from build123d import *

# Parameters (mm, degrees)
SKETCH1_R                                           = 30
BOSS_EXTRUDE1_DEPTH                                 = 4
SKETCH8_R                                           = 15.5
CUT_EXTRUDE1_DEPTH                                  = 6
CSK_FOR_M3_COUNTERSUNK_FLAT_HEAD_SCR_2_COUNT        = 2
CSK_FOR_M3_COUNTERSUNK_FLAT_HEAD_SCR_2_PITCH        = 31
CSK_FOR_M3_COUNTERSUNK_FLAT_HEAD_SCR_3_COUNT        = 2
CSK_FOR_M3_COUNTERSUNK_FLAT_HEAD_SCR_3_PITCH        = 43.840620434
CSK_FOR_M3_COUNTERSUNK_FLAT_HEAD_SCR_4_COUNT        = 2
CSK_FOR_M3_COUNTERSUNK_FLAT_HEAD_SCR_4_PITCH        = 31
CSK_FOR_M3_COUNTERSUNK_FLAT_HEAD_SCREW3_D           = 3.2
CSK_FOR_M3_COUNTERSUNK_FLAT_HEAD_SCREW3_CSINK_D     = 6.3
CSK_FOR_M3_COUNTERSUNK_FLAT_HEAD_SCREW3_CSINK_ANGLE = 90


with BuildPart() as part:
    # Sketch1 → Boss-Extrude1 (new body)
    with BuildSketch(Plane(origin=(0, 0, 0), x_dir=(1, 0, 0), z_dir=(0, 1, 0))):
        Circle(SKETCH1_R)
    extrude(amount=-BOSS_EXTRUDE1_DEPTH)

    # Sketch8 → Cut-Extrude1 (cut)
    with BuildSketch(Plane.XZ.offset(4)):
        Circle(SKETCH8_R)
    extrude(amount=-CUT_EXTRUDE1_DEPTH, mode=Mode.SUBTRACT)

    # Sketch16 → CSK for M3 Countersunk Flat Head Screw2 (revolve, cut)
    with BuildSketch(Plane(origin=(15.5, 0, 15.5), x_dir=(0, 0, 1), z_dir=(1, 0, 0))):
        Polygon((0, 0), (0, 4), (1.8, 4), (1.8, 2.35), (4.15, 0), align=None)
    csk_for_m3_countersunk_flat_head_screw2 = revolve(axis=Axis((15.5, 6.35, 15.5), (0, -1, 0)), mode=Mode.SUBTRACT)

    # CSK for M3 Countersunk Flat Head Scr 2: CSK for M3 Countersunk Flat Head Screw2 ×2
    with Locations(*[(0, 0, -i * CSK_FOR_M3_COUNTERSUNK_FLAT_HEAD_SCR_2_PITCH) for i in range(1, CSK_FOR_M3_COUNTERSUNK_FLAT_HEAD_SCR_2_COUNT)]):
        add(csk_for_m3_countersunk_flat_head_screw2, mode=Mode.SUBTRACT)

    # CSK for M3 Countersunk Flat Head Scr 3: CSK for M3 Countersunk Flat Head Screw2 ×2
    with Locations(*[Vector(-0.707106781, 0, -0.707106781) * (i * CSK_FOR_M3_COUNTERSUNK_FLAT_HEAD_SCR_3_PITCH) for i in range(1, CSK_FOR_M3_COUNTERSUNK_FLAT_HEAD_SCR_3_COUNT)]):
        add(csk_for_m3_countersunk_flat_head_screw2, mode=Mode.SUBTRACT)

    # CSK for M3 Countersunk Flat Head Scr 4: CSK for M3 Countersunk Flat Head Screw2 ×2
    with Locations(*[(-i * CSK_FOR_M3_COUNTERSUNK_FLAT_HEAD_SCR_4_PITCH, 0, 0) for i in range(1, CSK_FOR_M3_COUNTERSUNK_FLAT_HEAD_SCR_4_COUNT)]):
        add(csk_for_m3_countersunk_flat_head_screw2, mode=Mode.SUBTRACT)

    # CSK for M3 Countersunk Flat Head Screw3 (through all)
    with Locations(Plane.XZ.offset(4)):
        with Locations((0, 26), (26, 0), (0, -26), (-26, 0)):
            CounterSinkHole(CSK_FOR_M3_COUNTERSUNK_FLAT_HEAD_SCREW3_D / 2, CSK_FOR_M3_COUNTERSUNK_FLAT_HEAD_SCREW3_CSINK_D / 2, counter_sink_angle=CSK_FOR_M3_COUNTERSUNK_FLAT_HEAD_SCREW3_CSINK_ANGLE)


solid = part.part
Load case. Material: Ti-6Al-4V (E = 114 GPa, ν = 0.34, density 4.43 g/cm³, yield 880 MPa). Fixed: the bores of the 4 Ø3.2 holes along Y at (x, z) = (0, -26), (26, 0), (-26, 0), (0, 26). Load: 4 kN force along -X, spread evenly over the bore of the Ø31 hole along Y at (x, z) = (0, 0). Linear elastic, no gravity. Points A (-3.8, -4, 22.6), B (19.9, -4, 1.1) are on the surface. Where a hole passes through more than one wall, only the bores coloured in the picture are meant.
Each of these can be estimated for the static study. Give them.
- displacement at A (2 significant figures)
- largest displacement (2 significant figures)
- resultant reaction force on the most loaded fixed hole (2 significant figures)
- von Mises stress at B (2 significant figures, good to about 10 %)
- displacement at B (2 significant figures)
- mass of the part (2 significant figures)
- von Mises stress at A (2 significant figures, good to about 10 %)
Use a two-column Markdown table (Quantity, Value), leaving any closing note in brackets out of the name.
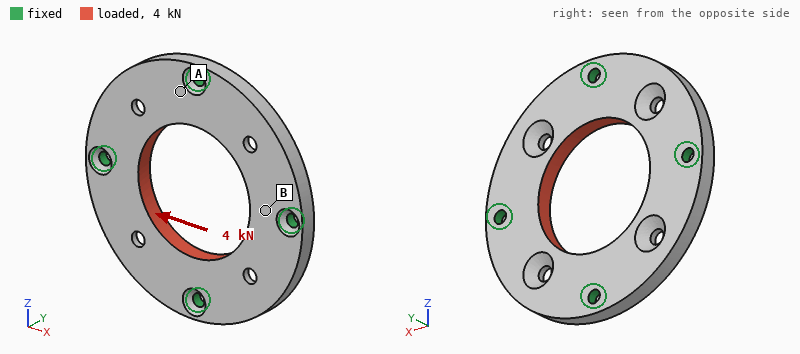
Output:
| Quantity | Value |
|---|---|
| displacement at A | 2.3 µm |
| largest displacement | 4.9 µm |
| resultant reaction force on the most loaded fixed hole | 1.0 kN |
| von Mises stress at B | 23 MPa |
| displacement at B | 2.1 µm |
| mass of the part | 34 g |
| von Mises stress at A | 11 MPa |
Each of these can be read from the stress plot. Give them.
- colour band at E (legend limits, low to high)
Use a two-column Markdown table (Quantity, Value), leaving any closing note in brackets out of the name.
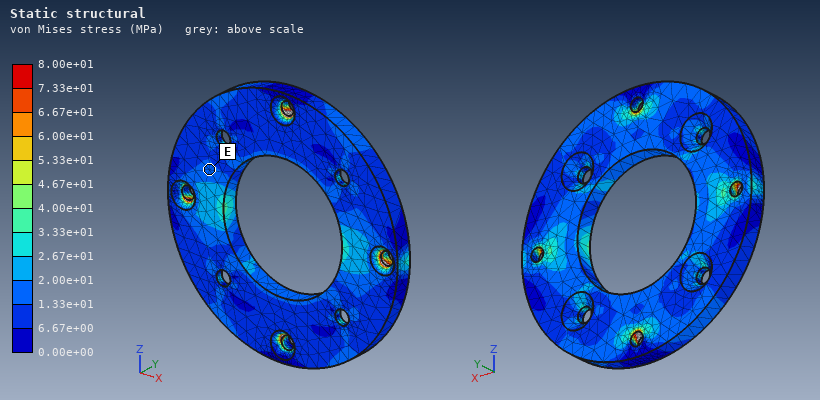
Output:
| Quantity | Value |
|---|---|
| colour band at E | 1.33e+01 to 2.00e+01 MPa |
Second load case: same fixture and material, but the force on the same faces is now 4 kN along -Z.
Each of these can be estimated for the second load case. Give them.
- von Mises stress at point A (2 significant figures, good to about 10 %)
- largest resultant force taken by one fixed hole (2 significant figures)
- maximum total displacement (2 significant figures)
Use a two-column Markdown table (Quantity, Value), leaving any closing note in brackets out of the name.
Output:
| Quantity | Value |
|---|---|
| von Mises stress at point A | 20 MPa |
| largest resultant force taken by one fixed hole | 1.0 kN |
| maximum total displacement | 4.9 µm |
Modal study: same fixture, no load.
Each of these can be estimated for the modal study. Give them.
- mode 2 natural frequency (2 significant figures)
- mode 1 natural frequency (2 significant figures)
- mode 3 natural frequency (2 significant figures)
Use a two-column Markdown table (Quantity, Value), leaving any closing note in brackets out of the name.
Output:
| Quantity | Value |
|---|---|
| mode 2 natural frequency | 11 kHz |
| mode 1 natural frequency | 9300 Hz |
| mode 3 natural frequency | 11 kHz |
